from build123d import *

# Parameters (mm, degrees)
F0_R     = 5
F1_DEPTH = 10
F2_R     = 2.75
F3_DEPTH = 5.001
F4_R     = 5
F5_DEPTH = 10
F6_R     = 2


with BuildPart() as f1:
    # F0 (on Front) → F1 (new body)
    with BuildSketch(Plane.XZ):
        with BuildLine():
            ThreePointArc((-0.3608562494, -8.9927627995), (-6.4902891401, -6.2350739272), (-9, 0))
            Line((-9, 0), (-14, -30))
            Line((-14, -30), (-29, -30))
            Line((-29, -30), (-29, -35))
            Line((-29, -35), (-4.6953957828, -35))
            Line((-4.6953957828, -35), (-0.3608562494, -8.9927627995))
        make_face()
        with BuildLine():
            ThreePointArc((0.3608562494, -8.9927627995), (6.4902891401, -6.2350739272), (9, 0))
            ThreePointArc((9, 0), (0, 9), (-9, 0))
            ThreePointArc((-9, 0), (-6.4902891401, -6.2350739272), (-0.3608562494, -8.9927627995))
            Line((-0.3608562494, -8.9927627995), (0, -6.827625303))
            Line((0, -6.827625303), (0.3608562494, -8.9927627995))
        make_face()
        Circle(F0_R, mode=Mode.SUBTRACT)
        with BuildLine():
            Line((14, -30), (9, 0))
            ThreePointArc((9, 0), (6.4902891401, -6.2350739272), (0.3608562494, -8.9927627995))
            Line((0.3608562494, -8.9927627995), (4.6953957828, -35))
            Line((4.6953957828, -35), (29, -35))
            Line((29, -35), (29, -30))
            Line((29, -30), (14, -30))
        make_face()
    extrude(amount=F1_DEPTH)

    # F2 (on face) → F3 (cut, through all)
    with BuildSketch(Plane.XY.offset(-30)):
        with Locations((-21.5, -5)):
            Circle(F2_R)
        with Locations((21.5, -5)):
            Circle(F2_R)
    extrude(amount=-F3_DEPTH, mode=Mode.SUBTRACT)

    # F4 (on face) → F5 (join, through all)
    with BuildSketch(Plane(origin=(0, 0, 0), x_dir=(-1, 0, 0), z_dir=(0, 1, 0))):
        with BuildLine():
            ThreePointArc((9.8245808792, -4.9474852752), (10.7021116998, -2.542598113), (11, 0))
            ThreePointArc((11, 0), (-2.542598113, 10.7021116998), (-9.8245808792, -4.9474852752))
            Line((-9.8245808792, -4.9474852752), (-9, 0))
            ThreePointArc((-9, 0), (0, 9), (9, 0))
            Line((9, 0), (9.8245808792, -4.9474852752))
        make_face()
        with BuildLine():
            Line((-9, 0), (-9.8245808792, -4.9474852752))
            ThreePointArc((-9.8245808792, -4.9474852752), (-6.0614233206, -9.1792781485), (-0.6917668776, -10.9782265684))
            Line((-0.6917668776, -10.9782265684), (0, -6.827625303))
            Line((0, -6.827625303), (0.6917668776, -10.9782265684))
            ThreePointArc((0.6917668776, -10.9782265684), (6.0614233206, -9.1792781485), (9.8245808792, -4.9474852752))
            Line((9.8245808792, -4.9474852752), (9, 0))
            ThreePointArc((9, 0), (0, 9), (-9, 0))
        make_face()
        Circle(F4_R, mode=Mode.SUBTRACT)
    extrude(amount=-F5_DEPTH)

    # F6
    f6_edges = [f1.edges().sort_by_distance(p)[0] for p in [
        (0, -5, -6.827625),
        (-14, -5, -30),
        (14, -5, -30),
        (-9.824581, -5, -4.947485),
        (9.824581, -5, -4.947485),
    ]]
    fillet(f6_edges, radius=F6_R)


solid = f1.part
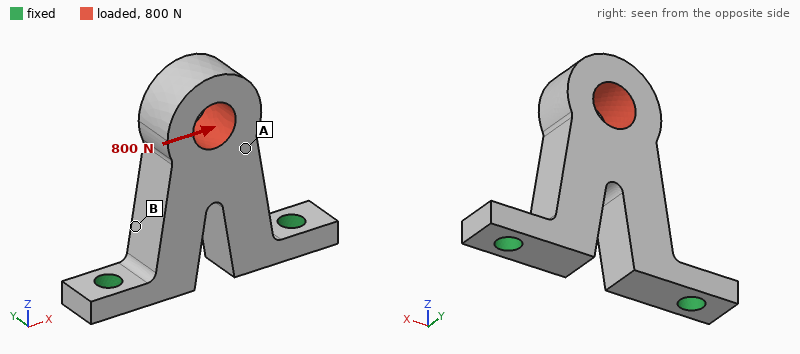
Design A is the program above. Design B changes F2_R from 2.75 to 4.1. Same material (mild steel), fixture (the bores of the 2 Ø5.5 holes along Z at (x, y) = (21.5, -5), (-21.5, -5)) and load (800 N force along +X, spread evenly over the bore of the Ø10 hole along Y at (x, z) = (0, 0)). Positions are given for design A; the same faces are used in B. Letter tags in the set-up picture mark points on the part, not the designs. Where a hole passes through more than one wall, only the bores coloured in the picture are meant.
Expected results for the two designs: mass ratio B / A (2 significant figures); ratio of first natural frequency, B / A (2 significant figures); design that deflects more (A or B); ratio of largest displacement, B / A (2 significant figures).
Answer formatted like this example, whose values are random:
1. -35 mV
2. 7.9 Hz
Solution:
1. 0.97
2. 1.1
3. A
4. 0.84
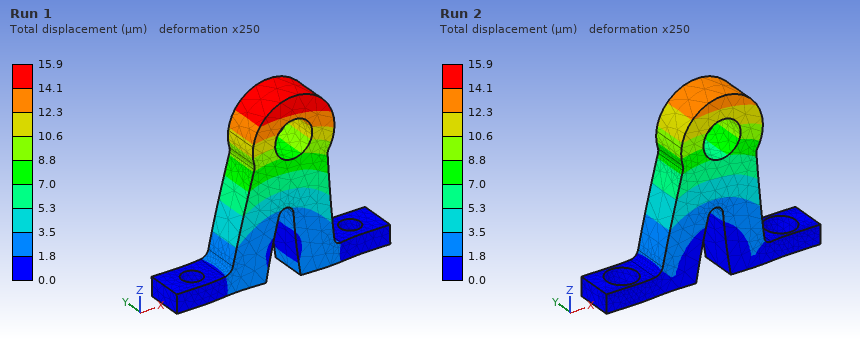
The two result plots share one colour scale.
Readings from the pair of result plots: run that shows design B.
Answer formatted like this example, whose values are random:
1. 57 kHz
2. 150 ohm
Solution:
1. Run 2
